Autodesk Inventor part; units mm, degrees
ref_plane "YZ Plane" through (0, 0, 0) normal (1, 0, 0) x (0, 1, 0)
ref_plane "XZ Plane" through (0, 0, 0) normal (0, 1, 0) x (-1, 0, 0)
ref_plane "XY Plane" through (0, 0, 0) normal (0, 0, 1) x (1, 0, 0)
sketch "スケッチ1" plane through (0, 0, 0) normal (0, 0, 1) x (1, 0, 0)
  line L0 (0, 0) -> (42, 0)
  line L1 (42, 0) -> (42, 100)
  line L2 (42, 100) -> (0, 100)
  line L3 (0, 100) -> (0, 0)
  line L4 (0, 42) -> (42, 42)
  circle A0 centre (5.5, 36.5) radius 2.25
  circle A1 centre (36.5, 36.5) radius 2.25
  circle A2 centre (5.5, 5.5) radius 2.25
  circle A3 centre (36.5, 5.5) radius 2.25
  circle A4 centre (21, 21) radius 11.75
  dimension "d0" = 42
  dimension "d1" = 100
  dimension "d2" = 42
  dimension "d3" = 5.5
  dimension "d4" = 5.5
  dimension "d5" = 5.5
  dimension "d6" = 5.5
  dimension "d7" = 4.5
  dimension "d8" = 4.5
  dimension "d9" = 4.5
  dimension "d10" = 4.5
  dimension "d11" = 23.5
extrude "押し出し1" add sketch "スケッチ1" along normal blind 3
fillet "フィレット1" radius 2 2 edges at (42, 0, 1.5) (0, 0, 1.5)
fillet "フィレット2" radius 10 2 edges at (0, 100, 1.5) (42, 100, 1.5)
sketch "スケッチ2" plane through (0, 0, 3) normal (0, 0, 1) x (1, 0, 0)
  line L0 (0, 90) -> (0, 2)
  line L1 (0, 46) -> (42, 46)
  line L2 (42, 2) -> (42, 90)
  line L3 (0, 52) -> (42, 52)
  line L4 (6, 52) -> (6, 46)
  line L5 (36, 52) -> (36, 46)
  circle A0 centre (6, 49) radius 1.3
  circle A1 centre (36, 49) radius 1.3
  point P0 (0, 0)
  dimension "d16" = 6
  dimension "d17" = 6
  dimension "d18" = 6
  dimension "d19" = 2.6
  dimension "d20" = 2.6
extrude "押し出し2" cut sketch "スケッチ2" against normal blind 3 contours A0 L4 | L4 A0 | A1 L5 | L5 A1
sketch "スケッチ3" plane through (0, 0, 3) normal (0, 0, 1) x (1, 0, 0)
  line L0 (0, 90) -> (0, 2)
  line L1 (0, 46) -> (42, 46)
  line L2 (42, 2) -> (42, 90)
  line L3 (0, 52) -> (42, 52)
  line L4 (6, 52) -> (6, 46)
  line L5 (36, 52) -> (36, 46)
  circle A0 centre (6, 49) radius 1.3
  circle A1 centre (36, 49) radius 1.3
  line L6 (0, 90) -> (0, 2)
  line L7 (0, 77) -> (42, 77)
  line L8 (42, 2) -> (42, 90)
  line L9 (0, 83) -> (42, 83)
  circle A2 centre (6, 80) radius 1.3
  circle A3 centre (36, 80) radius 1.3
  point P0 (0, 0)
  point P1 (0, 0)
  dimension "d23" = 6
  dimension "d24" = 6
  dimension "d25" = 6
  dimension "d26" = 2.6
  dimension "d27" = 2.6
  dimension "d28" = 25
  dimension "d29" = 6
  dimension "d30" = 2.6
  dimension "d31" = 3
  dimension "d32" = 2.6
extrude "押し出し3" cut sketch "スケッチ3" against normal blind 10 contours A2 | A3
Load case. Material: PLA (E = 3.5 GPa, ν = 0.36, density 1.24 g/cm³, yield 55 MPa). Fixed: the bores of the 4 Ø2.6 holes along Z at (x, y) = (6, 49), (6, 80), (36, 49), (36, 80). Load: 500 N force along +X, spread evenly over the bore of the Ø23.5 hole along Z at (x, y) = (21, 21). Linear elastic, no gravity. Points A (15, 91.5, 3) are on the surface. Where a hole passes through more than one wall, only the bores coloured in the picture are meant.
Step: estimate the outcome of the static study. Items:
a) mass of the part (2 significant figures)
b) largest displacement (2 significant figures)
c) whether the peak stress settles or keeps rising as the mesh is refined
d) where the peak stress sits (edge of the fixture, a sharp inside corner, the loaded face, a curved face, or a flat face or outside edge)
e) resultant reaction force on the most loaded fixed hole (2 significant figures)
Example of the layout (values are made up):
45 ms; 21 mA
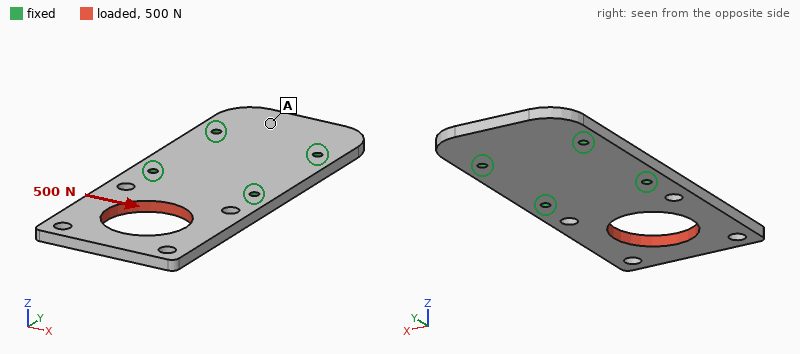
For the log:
14 g; 0.57 mm; keeps rising; edge of the fixture; 470 N
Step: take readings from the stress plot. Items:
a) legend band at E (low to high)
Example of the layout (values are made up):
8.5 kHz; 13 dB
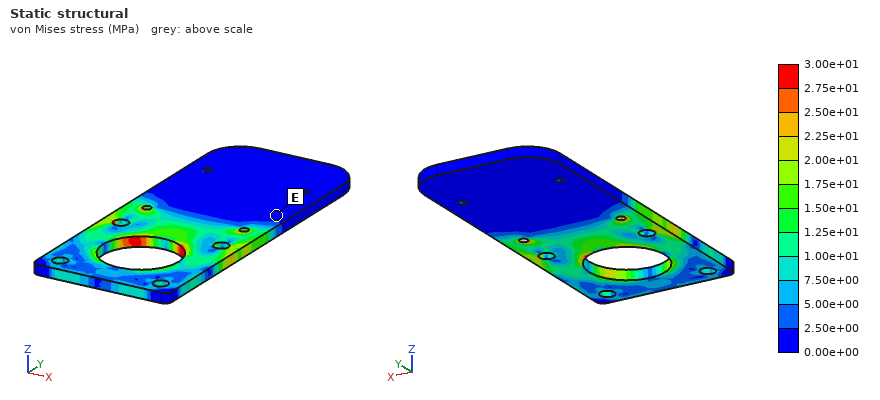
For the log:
0.00e+00 to 2.50e+00 MPa
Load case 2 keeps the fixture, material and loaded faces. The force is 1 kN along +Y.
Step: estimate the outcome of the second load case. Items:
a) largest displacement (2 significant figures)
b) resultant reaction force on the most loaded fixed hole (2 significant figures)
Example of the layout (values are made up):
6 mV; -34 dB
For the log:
0.23 mm; 420 N
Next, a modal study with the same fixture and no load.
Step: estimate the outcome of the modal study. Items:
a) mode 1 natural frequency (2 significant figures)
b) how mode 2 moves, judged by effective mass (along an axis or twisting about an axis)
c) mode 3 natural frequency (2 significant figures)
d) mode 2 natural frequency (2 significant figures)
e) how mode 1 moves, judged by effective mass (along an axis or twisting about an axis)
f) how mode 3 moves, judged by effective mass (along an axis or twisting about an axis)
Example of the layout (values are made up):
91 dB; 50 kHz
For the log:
320 Hz; twisting about Y; 1800 Hz; 800 Hz; along Z; along Z
